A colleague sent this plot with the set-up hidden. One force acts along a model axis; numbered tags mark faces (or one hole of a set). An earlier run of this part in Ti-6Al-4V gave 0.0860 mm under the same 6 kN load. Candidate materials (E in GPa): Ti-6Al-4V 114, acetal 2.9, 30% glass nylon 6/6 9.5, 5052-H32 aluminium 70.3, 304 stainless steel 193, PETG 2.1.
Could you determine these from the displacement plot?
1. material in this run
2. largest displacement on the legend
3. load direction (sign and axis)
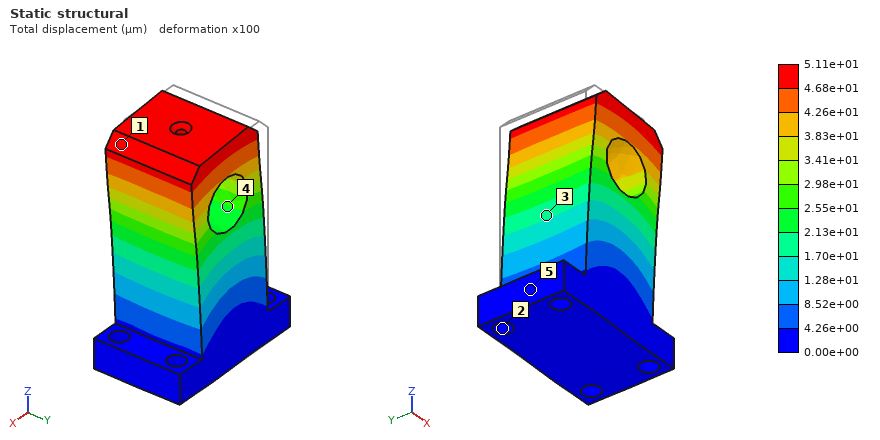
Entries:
304 stainless steel
5.11e+01 µm
+X
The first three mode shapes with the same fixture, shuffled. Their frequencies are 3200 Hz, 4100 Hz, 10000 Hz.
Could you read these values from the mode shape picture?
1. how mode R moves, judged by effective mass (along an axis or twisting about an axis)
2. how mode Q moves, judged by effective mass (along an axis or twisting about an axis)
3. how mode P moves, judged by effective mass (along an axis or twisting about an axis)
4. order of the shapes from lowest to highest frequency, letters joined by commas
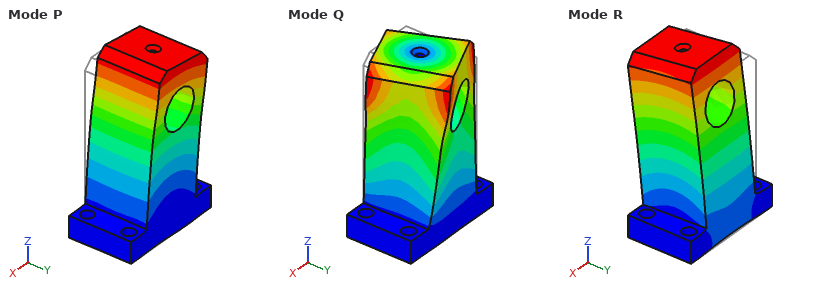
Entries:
along Y
twisting about Z
along X
R, P, Q
